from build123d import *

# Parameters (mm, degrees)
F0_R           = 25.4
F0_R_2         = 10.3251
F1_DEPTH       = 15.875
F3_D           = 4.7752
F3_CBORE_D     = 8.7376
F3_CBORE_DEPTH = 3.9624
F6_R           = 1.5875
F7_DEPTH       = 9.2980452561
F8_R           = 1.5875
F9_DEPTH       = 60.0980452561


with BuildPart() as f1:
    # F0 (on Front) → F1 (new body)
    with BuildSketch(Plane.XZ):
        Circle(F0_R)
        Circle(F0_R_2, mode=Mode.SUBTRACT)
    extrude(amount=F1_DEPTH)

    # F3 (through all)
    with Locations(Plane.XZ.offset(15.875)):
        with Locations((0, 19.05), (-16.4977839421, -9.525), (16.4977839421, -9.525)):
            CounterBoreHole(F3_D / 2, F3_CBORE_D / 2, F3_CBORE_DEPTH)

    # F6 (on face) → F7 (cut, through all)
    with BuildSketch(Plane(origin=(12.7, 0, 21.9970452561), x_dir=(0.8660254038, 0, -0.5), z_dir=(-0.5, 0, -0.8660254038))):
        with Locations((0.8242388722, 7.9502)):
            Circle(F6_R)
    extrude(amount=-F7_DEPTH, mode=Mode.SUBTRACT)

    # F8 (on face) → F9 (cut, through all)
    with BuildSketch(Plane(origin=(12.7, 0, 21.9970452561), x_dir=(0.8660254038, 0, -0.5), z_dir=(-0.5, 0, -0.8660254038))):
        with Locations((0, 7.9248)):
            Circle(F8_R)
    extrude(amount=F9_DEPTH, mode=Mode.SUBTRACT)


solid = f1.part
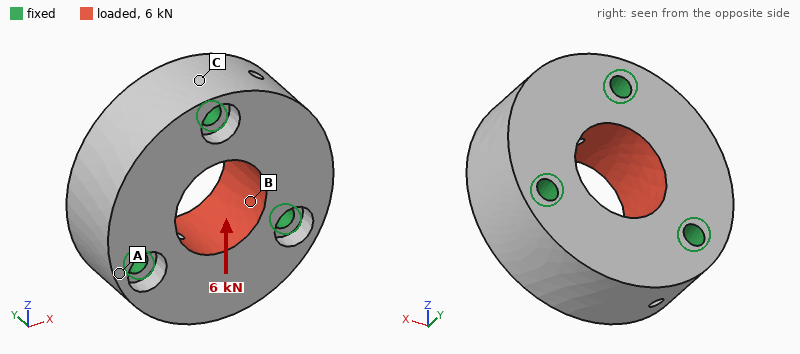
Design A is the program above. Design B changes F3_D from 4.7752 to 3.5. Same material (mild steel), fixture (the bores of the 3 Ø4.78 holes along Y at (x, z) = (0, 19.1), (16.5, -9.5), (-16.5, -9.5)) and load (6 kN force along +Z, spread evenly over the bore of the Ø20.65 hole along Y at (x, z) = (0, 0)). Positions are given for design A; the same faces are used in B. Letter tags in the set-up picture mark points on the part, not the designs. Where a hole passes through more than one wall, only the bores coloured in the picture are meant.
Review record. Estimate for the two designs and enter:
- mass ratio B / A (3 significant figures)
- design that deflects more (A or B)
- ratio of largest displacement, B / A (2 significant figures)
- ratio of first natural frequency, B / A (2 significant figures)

1.01
B
1.1
0.92
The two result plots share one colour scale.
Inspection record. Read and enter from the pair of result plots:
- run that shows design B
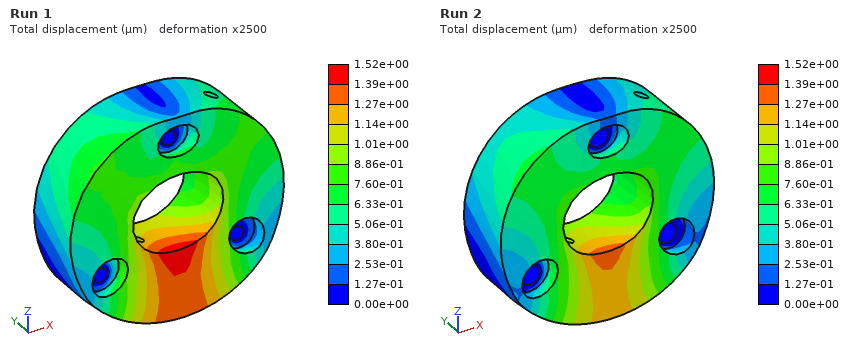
Run 1
